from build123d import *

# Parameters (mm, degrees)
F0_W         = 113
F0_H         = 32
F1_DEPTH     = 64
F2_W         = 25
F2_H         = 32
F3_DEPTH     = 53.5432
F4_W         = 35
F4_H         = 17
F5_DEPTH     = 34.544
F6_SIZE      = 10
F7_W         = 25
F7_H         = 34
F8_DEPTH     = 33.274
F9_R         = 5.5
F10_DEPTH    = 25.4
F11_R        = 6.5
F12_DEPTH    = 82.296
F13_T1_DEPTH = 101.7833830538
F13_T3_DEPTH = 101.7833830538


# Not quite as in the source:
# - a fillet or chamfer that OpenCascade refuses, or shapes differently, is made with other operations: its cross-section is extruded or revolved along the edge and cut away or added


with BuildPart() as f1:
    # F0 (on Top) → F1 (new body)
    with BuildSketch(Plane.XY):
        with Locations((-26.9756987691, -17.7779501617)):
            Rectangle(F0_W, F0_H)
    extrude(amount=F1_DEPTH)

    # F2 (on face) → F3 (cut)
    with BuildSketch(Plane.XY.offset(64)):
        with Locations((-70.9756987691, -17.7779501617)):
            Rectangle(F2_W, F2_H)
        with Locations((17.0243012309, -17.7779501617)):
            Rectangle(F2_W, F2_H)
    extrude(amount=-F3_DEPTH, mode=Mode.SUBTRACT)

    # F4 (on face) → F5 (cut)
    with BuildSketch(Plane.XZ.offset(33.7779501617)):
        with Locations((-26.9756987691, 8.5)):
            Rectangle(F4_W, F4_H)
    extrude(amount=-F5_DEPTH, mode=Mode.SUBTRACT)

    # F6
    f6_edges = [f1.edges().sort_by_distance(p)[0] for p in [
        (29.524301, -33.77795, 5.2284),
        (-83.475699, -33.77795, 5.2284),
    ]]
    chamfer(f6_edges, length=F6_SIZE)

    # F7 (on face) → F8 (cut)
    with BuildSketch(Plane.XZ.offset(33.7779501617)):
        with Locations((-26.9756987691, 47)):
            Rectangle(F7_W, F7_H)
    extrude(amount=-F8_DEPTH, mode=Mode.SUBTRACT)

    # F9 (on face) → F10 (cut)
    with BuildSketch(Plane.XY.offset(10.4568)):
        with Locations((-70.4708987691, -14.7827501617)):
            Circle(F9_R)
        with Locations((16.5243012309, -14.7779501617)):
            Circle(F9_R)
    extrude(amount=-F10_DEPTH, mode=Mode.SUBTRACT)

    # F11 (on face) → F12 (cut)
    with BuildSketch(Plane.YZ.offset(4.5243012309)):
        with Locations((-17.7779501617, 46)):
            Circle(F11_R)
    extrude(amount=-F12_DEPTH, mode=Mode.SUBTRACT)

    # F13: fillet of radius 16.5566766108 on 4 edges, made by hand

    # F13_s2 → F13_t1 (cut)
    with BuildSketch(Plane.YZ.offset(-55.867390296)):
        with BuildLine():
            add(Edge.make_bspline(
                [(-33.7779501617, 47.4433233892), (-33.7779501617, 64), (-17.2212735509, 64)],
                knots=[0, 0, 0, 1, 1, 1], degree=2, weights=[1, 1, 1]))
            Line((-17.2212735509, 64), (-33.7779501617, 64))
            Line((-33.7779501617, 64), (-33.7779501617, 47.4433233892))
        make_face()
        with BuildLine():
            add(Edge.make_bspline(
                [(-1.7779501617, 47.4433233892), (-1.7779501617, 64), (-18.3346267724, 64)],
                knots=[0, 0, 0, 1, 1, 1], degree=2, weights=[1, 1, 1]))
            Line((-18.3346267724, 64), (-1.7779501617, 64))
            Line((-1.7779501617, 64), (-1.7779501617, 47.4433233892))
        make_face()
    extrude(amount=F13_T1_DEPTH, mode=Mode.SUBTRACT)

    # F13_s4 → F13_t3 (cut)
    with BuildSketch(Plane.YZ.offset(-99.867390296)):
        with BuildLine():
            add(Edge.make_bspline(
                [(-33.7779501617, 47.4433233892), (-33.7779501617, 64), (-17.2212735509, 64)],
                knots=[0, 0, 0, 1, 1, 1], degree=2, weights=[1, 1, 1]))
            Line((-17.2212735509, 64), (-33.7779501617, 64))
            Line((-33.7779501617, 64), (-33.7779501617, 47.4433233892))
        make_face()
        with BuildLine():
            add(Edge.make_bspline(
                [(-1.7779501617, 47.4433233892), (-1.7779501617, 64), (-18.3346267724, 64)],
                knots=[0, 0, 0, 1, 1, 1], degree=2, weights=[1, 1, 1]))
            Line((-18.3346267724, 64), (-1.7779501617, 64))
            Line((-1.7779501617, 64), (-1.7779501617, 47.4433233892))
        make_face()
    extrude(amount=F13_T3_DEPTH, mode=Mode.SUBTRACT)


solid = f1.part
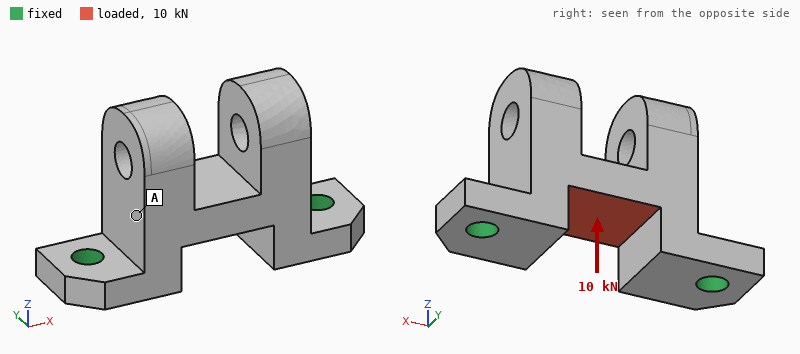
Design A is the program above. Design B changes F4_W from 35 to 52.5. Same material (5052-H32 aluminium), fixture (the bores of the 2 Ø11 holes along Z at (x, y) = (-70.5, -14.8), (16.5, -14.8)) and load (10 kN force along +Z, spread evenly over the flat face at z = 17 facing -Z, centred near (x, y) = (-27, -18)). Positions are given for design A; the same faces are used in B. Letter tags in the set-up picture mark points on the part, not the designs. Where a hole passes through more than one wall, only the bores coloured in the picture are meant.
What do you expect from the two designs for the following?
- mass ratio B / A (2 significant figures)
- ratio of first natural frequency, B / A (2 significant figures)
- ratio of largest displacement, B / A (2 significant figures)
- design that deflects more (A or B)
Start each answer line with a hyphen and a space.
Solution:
- 0.89
- 0.96
- 1.6
- B
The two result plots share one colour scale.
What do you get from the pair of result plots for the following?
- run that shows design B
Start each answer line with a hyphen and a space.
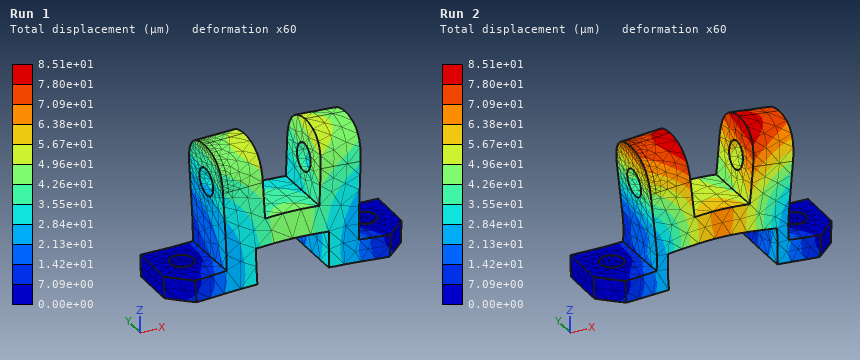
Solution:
- Run 2
